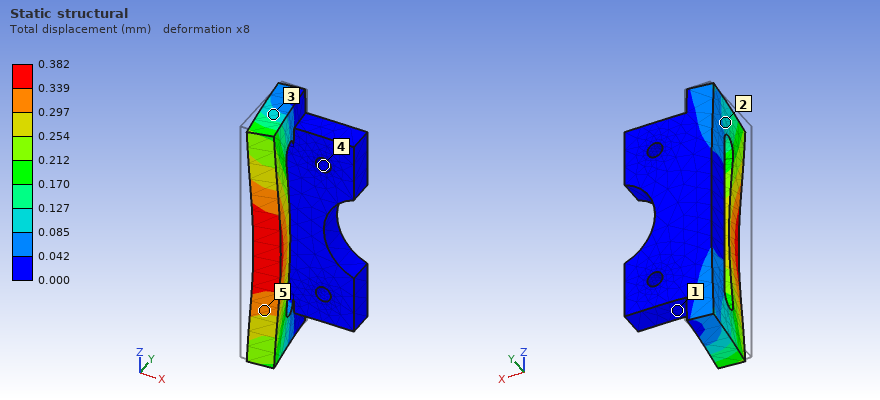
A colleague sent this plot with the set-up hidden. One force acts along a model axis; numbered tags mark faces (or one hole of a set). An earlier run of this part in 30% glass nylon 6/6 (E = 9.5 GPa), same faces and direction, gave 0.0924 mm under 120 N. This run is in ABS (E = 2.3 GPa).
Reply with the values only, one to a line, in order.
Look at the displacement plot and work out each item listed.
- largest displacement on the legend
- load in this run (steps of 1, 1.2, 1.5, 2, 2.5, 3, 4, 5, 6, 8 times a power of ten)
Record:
0.382 mm
120 N
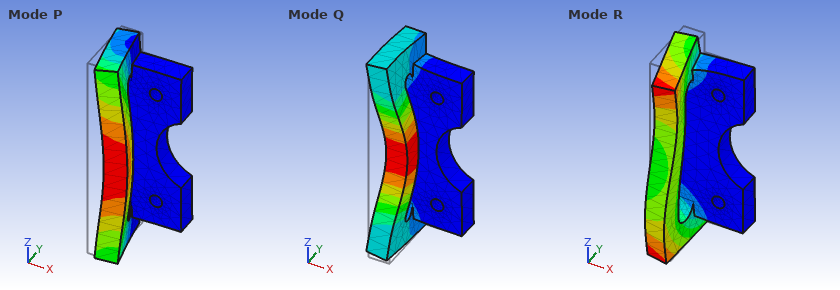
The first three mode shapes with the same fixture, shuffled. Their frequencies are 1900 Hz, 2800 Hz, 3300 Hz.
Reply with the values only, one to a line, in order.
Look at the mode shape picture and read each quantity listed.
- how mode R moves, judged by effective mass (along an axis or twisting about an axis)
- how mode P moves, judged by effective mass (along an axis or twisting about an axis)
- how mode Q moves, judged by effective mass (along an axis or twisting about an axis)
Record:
along Z
along X
along Y
